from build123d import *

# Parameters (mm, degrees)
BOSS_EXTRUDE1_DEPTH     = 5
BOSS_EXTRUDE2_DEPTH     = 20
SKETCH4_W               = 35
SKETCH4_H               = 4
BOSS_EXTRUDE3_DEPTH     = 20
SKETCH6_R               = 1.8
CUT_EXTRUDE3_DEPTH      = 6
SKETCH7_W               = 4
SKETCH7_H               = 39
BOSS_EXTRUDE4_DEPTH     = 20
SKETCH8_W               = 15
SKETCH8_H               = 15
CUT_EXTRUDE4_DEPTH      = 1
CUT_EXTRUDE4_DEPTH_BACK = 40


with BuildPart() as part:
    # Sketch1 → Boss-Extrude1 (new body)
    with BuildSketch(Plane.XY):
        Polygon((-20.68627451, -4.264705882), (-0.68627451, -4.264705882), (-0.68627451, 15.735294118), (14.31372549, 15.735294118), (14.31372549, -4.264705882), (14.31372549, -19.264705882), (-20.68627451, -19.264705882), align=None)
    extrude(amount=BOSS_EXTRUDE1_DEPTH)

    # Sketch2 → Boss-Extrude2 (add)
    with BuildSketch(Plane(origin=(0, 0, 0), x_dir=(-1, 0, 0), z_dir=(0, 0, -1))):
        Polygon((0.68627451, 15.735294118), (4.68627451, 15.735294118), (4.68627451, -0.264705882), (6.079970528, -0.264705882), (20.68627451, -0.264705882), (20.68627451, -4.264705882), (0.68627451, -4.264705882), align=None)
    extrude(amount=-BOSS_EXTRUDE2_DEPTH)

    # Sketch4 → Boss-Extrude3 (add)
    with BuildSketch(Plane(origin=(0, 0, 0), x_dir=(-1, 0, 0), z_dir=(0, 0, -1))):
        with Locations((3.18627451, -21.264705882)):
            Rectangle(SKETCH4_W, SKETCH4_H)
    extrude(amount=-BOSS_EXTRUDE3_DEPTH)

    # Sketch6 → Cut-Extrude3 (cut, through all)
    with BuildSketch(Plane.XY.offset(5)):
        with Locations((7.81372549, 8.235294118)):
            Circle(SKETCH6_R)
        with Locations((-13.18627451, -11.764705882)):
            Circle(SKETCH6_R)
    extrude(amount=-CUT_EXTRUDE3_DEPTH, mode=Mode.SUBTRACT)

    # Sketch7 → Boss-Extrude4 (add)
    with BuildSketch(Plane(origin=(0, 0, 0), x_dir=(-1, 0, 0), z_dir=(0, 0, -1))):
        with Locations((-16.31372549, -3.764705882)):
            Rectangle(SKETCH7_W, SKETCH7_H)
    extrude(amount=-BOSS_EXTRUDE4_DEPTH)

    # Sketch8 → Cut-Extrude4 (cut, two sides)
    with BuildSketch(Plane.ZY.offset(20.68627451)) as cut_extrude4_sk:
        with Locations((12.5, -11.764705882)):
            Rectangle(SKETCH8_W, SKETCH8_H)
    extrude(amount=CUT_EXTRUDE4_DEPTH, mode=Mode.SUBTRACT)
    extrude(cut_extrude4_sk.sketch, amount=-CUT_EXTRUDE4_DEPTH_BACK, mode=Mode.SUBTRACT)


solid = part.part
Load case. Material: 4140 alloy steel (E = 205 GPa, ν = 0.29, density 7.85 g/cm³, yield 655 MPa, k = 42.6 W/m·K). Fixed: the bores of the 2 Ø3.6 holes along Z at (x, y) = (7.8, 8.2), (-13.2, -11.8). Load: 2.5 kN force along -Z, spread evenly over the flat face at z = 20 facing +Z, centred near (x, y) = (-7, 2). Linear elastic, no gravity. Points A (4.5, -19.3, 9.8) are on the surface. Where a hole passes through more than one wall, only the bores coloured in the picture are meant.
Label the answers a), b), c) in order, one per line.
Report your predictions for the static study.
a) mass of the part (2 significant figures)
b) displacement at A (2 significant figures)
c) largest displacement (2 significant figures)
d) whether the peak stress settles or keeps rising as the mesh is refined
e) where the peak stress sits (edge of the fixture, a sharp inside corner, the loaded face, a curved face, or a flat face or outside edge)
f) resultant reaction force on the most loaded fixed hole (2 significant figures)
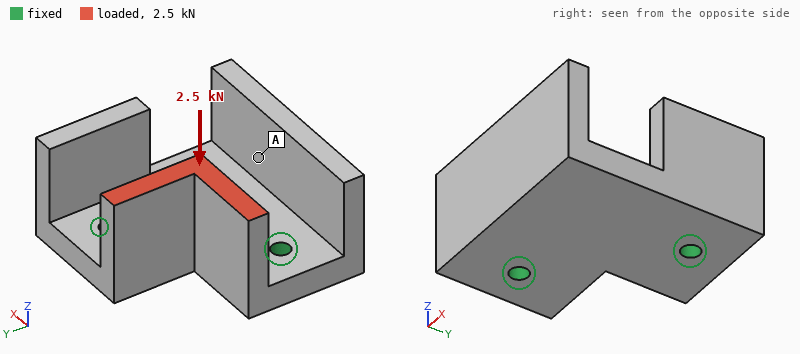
a) 94 g
b) 4.4 µm
c) 23 µm
d) keeps rising
e) edge of the fixture
f) 1.3 kN
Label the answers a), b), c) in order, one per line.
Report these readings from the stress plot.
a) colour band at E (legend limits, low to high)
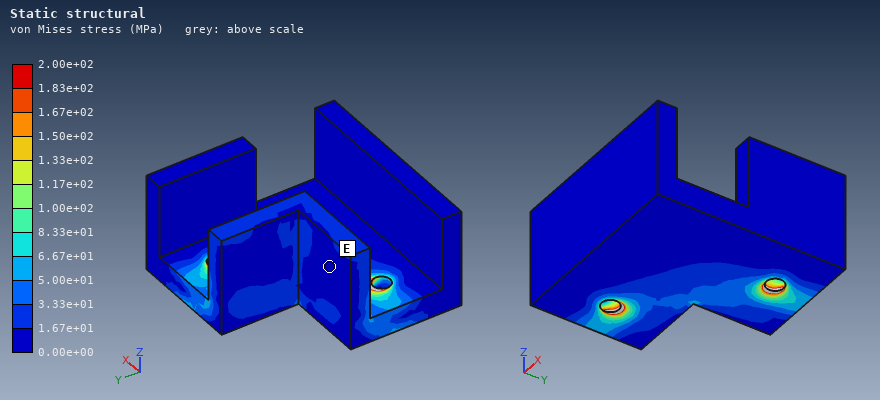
a) 0.00e+00 to 1.67e+01 MPa
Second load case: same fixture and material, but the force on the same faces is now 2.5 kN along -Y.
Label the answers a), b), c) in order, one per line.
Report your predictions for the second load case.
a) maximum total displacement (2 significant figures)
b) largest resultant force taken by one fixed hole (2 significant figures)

a) 94 µm
b) 1.8 kN
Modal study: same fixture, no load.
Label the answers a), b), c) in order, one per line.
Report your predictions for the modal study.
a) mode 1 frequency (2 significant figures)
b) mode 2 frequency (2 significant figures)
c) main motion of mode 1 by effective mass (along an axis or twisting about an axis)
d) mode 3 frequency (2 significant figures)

a) 4500 Hz
b) 7500 Hz
c) along Z
d) 8400 Hz
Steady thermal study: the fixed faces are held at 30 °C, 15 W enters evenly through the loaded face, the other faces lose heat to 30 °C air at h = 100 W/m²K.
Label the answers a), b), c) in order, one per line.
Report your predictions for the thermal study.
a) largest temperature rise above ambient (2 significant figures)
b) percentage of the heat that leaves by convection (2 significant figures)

a) 47 K
b) 37 %
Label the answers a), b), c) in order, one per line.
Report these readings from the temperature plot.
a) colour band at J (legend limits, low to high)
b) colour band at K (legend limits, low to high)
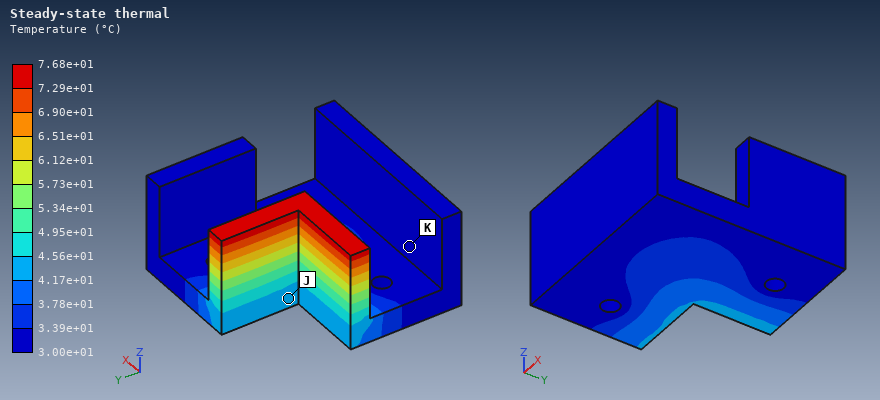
a) 4.17e+01 to 4.56e+01 °C
b) 3.00e+01 to 3.39e+01 °C
